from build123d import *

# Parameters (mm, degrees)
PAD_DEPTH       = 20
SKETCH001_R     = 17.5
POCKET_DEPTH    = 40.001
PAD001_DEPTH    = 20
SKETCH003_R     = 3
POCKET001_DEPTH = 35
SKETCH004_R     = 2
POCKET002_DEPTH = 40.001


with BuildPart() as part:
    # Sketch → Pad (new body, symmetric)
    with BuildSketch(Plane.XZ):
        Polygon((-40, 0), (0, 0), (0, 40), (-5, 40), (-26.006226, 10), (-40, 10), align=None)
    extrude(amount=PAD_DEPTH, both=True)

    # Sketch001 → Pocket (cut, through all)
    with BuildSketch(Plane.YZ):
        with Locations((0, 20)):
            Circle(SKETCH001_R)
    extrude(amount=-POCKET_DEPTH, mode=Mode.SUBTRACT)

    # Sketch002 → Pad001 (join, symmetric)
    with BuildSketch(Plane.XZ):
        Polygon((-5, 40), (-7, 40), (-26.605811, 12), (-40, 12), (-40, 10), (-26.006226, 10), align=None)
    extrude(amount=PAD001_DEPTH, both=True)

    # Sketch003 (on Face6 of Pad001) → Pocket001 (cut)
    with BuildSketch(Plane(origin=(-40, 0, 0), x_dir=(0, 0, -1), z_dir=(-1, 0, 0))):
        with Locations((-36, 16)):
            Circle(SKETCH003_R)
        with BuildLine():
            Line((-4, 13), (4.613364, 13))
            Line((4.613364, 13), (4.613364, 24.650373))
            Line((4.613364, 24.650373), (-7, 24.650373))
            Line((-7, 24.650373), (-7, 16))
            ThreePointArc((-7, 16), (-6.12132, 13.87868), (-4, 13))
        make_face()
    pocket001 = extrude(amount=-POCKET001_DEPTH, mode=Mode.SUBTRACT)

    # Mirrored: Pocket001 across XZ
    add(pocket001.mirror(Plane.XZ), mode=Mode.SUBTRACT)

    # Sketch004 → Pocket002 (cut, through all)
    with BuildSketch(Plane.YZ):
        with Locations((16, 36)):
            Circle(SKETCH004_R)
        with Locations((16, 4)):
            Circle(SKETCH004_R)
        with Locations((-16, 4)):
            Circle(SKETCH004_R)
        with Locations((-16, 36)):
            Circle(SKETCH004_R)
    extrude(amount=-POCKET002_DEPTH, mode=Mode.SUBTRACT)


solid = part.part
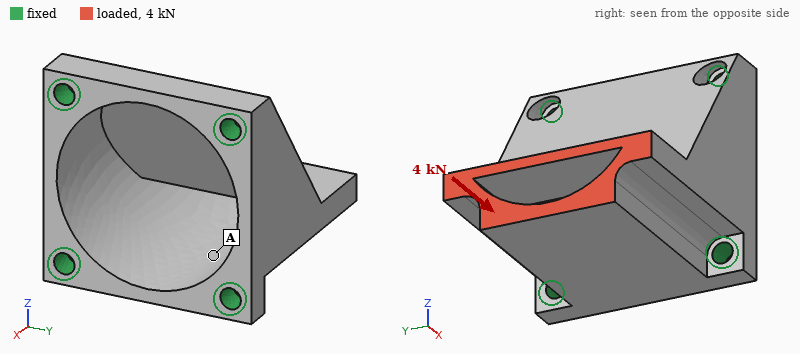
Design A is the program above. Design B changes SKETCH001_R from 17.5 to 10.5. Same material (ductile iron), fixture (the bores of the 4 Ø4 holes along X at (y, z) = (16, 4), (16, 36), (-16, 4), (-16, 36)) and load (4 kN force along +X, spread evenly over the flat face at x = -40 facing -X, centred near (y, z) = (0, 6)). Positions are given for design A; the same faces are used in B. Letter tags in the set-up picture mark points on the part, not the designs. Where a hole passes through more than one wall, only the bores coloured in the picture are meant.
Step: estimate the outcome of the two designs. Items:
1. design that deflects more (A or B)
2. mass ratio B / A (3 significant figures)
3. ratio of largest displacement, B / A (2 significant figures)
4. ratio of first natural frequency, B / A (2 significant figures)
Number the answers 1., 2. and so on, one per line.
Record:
1. A
2. 1.95
3. 0.60
4. 1.1
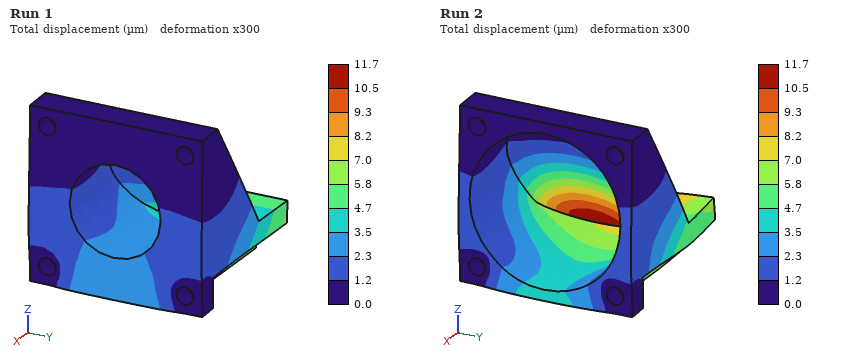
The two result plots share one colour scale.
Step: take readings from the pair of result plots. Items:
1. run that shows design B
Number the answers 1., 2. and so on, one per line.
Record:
1. Run 1
